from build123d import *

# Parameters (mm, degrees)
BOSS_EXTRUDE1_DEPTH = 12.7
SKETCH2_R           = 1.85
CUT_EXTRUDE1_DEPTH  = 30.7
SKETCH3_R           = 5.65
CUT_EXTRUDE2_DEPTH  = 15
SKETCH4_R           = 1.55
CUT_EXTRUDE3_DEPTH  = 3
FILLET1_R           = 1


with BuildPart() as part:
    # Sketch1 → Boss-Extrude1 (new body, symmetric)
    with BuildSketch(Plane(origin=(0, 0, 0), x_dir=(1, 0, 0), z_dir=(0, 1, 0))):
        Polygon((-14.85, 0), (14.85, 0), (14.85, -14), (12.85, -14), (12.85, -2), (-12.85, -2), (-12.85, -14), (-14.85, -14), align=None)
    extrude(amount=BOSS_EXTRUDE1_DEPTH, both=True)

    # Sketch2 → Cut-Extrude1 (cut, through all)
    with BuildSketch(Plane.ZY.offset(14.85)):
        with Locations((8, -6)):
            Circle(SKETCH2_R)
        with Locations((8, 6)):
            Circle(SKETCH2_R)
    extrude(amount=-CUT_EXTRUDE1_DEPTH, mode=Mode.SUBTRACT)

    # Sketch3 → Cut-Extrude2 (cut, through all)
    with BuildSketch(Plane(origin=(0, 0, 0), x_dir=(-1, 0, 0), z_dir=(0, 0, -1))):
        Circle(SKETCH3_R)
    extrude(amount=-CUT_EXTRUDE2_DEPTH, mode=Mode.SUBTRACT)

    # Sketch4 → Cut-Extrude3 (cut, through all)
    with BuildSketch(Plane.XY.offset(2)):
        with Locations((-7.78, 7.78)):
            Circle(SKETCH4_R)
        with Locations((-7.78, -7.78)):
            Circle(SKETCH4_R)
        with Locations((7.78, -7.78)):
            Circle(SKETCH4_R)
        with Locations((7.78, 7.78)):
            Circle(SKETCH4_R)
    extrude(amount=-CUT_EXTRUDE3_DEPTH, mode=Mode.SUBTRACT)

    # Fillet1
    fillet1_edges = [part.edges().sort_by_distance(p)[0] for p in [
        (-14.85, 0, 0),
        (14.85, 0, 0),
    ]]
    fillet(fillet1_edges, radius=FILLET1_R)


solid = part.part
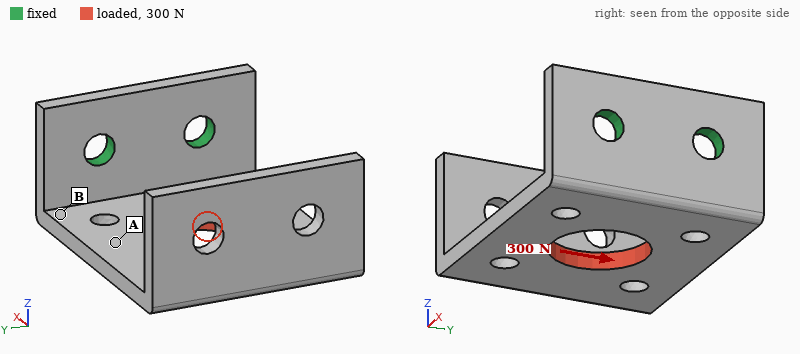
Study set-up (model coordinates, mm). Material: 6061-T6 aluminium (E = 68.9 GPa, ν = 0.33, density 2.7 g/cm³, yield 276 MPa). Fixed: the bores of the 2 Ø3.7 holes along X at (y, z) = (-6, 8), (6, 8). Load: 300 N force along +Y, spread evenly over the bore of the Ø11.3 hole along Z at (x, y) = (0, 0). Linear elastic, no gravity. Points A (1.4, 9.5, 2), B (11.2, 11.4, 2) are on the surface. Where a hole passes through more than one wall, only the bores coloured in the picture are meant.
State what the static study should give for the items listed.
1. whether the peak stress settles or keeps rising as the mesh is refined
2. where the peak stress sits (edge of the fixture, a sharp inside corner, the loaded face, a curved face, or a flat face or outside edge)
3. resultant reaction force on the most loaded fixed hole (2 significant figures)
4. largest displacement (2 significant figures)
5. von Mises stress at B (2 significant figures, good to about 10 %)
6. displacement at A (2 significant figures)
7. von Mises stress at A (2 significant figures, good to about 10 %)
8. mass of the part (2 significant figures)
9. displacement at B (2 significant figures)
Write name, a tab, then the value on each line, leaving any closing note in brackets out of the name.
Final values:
whether the peak stress settles or keeps rising as the mesh is refined	keeps rising
where the peak stress sits	edge of the fixture
resultant reaction force on the most loaded fixed hole	330 N
largest displacement	0.17 mm
von Mises stress at B	54 MPa
displacement at A	0.070 mm
von Mises stress at A	25 MPa
mass of the part	6.4 g
displacement at B	0.040 mm
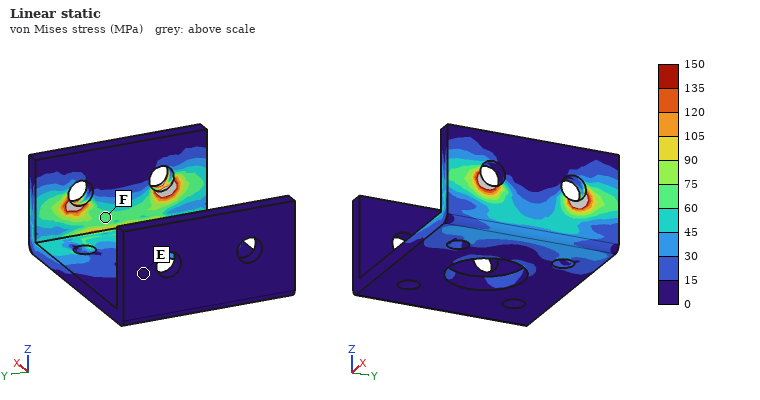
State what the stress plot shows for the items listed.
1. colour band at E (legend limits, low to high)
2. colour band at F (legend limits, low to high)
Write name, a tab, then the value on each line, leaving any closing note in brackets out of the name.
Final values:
colour band at E	0 to 15 MPa
colour band at F	60 to 75 MPa
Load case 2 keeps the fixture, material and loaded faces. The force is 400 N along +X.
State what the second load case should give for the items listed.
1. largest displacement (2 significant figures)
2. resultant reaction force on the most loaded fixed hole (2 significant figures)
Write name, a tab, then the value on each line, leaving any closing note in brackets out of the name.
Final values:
largest displacement	0.18 mm
resultant reaction force on the most loaded fixed hole	200 N
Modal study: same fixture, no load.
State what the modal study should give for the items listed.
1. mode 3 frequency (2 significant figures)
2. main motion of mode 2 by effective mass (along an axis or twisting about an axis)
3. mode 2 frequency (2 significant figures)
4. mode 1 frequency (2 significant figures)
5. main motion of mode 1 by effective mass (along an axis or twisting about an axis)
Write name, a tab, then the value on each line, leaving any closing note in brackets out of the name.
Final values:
mode 3 frequency	4000 Hz
main motion of mode 2 by effective mass	along Y
mode 2 frequency	2100 Hz
mode 1 frequency	900 Hz
main motion of mode 1 by effective mass	along Z
